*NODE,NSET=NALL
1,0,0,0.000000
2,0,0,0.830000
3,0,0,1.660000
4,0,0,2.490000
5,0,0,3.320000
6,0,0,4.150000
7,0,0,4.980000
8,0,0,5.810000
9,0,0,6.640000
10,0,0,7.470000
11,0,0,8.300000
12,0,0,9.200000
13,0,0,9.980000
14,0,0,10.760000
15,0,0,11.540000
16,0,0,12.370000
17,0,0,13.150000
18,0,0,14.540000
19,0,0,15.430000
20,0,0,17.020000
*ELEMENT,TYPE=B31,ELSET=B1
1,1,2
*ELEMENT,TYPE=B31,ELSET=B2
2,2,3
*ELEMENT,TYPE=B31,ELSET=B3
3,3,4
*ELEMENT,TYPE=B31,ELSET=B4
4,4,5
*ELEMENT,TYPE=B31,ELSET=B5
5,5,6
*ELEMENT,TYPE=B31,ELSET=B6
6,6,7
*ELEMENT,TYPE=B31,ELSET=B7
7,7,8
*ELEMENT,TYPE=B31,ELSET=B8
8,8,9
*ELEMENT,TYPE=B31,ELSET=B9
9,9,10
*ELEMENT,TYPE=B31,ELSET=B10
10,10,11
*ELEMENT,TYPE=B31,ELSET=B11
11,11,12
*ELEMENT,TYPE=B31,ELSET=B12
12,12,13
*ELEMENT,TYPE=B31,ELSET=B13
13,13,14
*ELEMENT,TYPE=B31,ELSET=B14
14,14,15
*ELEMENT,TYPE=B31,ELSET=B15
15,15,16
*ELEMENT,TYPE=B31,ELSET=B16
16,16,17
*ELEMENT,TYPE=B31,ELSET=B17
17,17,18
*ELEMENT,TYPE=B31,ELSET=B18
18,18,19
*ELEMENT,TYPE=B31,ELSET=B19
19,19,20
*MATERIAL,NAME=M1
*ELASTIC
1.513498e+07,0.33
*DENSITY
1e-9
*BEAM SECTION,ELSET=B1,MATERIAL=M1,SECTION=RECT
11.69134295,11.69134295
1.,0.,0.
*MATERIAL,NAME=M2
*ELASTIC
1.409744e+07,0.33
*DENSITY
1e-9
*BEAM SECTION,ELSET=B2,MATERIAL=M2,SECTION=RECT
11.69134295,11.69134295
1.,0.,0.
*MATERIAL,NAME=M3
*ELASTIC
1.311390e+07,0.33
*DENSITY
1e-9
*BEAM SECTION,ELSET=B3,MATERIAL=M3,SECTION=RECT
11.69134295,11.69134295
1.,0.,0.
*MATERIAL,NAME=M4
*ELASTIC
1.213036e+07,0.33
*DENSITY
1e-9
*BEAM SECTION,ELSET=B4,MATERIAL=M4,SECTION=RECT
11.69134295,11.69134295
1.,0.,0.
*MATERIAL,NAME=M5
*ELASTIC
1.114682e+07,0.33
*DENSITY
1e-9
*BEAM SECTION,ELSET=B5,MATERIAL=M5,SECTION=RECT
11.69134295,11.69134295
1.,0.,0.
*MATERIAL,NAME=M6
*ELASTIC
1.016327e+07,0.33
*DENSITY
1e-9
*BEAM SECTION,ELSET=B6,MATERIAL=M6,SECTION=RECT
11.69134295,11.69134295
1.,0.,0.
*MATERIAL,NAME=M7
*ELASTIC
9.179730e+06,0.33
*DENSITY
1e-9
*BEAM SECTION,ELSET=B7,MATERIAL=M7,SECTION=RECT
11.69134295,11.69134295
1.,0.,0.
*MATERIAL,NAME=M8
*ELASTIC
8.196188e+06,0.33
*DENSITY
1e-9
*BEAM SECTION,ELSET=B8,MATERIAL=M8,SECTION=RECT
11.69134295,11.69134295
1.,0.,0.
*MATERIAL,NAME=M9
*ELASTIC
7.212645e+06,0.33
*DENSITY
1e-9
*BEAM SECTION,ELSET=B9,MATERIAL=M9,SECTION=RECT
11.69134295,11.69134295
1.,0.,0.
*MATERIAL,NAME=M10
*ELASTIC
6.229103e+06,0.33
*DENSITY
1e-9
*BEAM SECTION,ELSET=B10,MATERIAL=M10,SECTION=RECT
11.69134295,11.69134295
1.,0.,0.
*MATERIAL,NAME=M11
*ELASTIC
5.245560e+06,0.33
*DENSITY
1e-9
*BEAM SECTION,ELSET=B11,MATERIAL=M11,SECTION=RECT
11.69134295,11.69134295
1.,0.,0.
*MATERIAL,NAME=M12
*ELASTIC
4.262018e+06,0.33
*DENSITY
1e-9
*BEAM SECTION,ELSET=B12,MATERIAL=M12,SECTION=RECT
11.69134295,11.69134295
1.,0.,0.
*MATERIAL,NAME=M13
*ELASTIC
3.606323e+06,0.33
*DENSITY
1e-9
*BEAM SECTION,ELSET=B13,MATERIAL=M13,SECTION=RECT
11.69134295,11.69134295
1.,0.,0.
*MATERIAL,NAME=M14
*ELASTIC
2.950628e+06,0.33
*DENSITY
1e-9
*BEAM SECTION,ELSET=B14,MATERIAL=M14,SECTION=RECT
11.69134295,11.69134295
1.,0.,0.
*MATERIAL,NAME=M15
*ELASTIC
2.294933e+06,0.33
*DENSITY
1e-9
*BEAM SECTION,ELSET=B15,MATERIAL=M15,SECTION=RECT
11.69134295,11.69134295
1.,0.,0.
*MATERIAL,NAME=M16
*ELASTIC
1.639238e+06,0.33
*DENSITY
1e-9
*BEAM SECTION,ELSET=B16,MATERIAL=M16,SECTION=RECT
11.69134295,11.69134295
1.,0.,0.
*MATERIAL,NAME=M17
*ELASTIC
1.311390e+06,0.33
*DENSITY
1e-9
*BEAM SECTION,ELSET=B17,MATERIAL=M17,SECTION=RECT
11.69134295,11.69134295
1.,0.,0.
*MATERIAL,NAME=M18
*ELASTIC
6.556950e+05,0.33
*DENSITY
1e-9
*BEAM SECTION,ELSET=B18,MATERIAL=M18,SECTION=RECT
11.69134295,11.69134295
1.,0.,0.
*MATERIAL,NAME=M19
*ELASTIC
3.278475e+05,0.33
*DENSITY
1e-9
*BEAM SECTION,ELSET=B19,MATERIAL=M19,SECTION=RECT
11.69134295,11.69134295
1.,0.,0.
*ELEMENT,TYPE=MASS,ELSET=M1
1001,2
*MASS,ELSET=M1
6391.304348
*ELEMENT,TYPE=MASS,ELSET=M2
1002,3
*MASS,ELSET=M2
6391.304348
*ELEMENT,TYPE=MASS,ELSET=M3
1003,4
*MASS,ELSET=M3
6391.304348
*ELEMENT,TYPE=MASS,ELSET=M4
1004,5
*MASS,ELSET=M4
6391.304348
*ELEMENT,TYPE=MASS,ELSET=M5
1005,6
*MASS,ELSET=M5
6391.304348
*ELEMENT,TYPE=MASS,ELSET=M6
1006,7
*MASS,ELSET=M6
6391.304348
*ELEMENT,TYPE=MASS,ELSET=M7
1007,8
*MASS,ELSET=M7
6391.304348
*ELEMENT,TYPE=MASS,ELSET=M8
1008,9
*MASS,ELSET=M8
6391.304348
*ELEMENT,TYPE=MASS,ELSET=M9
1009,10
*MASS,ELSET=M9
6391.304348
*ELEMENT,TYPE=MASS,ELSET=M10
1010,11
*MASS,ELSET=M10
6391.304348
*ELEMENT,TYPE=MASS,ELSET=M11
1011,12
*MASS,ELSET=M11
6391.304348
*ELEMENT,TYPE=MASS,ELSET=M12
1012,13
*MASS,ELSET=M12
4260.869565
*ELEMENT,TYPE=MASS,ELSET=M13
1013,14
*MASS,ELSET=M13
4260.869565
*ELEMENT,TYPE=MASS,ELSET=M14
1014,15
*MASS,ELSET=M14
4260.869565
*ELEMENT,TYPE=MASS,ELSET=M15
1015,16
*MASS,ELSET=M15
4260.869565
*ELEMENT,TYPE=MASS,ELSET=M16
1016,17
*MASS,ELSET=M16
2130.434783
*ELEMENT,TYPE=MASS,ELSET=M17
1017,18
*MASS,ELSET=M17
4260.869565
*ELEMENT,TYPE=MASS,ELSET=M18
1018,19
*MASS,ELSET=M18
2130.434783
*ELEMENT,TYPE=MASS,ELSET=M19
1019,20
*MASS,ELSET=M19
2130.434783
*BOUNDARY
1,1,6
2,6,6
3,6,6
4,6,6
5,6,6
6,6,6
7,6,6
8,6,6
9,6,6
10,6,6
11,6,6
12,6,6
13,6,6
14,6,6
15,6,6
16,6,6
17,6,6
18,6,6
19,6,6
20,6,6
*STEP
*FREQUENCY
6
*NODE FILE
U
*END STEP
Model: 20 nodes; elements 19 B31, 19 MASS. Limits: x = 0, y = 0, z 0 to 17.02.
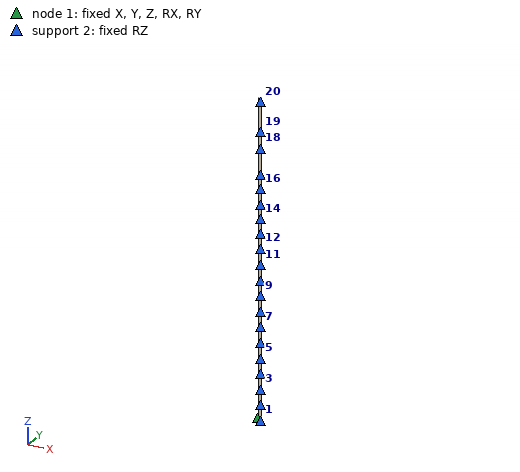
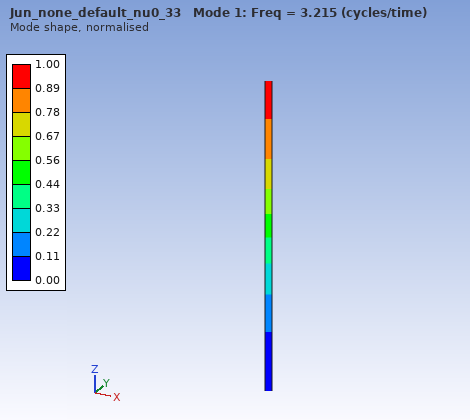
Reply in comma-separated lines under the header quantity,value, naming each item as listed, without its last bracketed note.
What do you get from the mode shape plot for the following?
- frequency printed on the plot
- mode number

quantity,value
frequency printed on the plot,3.215
mode number,1
